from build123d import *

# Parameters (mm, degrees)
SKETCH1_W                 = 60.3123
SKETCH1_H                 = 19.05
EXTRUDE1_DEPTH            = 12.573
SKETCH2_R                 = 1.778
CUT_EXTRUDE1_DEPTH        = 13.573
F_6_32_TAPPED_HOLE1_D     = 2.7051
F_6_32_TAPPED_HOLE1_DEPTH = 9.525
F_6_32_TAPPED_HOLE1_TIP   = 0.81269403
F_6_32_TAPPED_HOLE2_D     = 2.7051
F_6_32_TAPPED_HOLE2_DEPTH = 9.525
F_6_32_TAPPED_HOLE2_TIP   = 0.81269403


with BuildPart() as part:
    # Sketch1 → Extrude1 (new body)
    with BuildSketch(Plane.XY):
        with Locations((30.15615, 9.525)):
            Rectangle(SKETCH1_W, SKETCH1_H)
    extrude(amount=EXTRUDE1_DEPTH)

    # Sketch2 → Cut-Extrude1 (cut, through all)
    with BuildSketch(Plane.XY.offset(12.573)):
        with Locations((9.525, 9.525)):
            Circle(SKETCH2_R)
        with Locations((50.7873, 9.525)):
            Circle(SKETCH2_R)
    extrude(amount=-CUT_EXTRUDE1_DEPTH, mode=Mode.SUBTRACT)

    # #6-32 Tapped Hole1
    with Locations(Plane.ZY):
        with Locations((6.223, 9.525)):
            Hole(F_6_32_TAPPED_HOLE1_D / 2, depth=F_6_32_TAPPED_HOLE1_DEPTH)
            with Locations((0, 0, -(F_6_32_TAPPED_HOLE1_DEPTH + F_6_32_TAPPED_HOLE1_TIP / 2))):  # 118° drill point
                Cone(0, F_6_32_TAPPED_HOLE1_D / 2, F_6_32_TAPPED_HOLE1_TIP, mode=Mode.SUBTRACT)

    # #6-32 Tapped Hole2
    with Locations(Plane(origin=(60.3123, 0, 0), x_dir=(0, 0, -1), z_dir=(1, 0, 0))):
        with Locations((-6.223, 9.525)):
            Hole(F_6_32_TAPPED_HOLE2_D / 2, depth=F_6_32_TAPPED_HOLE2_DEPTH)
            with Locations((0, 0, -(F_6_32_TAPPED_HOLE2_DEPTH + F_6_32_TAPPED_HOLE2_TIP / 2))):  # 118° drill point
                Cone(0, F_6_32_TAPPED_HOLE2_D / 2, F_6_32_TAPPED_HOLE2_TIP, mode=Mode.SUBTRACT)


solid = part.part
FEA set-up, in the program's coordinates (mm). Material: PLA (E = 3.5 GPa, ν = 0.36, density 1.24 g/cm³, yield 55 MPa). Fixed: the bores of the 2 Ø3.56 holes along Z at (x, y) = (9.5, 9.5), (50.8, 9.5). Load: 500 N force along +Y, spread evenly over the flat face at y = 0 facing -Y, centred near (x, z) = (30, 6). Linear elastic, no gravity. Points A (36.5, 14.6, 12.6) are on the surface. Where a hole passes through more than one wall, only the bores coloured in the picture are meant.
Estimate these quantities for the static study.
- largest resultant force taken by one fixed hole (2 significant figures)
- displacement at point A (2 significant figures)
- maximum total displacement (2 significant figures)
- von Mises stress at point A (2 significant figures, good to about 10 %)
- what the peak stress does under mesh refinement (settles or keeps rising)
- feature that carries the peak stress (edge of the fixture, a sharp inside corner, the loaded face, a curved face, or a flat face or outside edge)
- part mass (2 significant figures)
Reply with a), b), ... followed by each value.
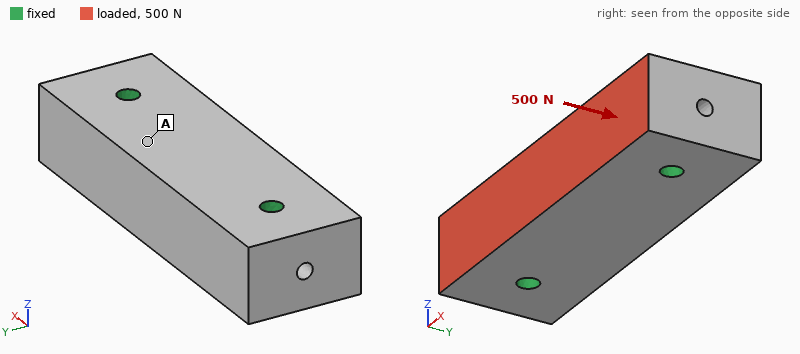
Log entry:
a) 250 N
b) 11 µm
c) 14 µm
d) 0.73 MPa
e) keeps rising
f) edge of the fixture
g) 17 g
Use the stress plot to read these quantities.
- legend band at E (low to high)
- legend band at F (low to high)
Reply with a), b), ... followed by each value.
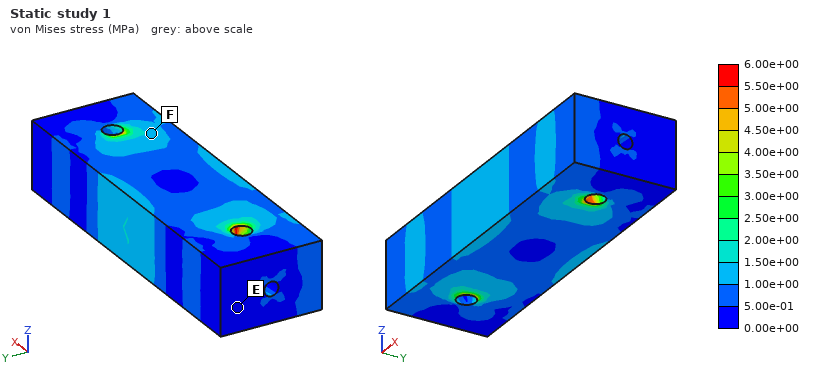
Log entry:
a) 0.00e+00 to 5.00e-01 MPa
b) 1.00e+00 to 1.50e+00 MPa
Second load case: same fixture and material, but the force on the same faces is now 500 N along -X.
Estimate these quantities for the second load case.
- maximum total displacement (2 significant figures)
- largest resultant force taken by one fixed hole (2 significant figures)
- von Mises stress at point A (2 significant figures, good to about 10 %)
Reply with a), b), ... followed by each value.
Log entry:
a) 15 µm
b) 270 N
c) 0.49 MPa
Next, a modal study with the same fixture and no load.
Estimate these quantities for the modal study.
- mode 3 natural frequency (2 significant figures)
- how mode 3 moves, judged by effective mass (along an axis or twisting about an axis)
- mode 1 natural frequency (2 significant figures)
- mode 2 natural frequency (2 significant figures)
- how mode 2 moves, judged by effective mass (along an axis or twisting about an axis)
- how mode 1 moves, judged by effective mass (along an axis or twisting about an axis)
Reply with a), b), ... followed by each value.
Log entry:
a) 9400 Hz
b) twisting about X
c) 7300 Hz
d) 7600 Hz
e) along Z
f) along Y
